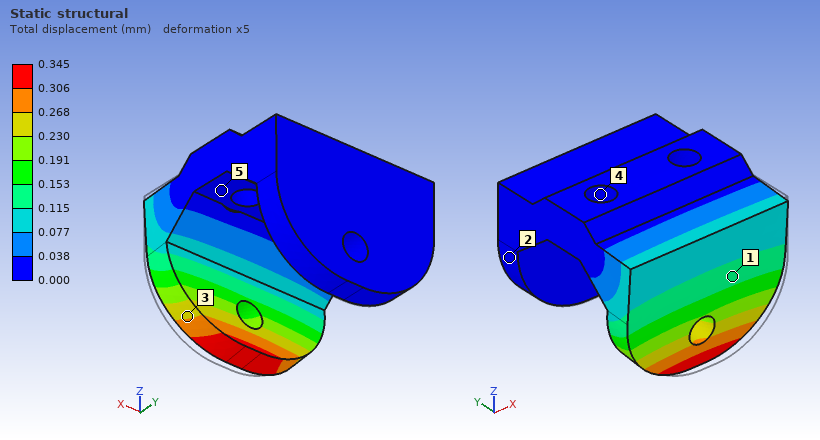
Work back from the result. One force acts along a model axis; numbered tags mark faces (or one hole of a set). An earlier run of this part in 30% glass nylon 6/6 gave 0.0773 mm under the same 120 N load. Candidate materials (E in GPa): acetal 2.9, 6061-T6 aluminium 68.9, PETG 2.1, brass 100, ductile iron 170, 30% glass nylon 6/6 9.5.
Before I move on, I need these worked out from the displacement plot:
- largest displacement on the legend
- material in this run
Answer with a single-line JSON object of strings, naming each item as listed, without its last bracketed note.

{"largest displacement on the legend": "0.345 mm", "material in this run": "PETG"}
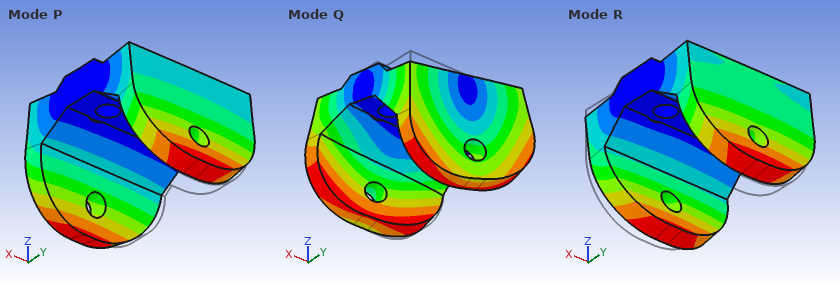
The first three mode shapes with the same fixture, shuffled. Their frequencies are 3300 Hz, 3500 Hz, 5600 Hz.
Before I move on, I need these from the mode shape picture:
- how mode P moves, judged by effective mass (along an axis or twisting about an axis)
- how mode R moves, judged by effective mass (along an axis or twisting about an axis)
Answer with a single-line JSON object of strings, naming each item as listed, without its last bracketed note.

{"how mode P moves, judged by effective mass": "along Z", "how mode R moves, judged by effective mass": "along Y"}
